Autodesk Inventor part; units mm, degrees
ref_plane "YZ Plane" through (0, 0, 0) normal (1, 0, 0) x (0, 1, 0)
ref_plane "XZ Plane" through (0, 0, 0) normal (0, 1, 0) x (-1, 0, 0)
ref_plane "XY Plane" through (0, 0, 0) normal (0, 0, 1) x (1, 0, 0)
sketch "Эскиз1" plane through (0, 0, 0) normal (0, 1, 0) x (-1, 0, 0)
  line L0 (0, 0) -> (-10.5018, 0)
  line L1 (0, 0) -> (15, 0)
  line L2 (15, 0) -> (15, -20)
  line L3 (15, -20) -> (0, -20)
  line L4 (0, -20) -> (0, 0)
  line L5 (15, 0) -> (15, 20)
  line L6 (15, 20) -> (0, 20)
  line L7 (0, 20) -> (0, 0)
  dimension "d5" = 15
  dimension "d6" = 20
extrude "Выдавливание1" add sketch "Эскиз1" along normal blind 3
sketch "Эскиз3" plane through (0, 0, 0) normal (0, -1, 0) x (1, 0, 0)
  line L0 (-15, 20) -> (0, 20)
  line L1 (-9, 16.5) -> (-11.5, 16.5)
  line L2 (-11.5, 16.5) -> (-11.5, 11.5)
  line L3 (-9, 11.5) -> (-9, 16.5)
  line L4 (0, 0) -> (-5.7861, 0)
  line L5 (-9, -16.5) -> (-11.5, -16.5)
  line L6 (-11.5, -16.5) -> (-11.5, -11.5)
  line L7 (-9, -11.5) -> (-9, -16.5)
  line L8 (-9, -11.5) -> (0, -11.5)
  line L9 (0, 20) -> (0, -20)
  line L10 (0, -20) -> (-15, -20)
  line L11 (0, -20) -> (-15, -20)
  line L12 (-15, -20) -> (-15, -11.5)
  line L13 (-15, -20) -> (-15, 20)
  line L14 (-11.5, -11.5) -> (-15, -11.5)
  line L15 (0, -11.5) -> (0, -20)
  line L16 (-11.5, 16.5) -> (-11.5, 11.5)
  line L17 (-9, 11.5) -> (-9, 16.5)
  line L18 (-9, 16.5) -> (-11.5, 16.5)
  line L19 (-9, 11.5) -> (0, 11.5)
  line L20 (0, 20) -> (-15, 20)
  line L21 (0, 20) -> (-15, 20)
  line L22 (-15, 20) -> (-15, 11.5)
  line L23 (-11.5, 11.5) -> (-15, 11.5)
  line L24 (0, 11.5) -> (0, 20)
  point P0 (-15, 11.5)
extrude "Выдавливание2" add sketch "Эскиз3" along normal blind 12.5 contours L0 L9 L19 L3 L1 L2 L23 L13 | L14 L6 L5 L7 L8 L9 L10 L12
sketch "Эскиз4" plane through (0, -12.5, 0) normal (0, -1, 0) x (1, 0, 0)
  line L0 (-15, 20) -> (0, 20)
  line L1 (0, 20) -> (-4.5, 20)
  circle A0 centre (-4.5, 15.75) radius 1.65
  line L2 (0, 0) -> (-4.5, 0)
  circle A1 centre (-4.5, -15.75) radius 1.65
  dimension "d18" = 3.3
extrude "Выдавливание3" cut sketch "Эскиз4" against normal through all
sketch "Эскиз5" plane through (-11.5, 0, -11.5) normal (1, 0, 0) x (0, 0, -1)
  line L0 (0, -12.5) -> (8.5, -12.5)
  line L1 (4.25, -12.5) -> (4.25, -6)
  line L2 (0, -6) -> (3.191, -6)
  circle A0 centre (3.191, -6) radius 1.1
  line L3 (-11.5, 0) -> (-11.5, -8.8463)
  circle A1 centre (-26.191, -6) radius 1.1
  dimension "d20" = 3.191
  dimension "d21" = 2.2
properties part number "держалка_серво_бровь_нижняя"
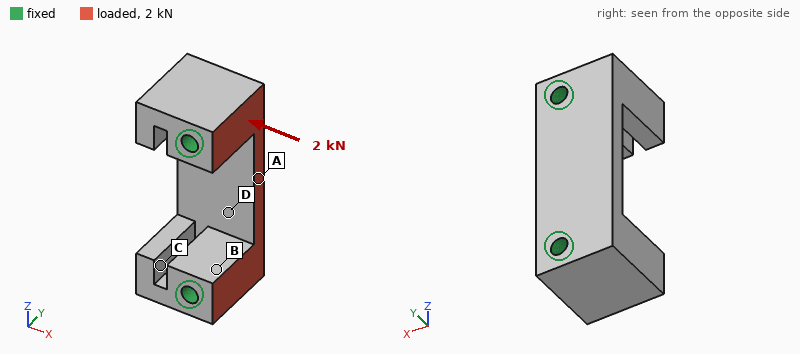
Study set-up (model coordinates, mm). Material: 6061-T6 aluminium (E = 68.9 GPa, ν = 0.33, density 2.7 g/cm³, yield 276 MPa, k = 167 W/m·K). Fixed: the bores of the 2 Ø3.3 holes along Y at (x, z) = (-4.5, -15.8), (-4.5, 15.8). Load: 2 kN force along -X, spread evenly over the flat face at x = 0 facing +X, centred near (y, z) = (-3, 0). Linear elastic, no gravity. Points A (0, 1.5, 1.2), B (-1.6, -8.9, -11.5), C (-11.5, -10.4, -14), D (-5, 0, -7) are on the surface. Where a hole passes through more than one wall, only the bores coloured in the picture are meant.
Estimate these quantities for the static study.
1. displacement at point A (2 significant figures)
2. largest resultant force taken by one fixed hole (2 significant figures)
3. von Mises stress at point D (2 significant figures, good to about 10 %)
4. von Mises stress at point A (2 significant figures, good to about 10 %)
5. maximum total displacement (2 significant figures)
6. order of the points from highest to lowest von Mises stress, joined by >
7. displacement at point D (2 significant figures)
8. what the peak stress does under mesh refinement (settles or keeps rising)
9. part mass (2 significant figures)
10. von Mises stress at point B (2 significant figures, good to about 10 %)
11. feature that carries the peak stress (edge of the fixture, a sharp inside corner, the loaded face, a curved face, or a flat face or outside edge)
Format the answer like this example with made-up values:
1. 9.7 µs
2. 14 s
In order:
1. 3.7 µm
2. 1.0 kN
3. 7.4 MPa
4. 9.7 MPa
5. 3.7 µm
6. A > D > B > C
7. 2.5 µm
8. keeps rising
9. 12 g
10. 5.0 MPa
11. edge of the fixture
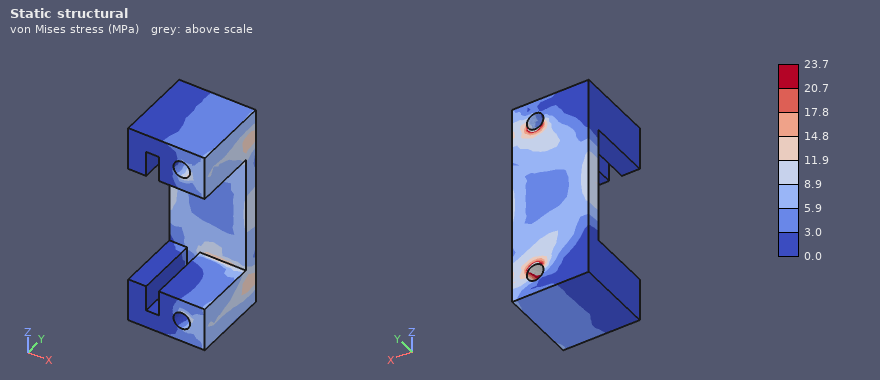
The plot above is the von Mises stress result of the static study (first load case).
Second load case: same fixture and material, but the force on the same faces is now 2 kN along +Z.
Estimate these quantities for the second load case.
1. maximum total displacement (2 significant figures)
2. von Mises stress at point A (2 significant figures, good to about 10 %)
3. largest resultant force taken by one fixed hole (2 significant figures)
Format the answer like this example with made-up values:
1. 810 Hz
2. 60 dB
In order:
1. 2.4 µm
2. 10 MPa
3. 1.0 kN
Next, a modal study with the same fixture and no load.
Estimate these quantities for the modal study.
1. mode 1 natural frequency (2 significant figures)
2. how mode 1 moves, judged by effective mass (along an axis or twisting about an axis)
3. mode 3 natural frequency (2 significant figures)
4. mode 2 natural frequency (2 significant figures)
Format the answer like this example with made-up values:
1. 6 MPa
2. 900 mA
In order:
1. 20 kHz
2. along Y
3. 32 kHz
4. 28 kHz
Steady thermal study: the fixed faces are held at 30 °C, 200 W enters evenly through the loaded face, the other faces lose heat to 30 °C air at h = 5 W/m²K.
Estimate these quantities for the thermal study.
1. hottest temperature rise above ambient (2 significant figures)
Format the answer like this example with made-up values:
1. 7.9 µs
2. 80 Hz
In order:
1. 44 K
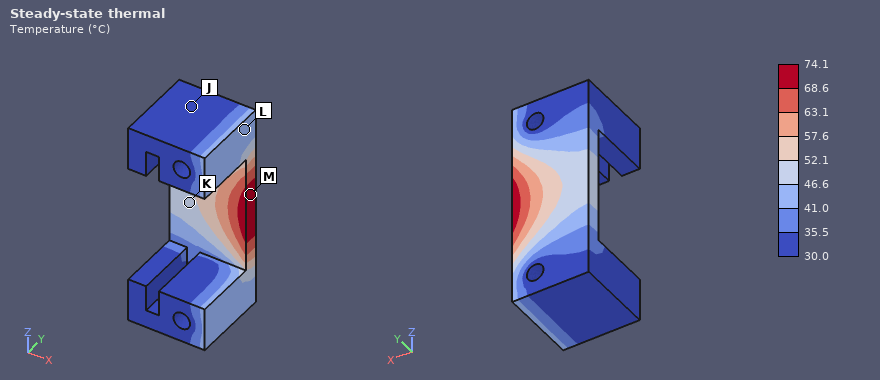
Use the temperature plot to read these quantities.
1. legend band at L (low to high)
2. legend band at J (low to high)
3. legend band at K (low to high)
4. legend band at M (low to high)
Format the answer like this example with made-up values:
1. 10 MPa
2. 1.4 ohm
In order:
1. 41.0 to 46.6 °C
2. 30.0 to 35.5 °C
3. 46.6 to 52.1 °C
4. 68.6 to 74.1 °C
